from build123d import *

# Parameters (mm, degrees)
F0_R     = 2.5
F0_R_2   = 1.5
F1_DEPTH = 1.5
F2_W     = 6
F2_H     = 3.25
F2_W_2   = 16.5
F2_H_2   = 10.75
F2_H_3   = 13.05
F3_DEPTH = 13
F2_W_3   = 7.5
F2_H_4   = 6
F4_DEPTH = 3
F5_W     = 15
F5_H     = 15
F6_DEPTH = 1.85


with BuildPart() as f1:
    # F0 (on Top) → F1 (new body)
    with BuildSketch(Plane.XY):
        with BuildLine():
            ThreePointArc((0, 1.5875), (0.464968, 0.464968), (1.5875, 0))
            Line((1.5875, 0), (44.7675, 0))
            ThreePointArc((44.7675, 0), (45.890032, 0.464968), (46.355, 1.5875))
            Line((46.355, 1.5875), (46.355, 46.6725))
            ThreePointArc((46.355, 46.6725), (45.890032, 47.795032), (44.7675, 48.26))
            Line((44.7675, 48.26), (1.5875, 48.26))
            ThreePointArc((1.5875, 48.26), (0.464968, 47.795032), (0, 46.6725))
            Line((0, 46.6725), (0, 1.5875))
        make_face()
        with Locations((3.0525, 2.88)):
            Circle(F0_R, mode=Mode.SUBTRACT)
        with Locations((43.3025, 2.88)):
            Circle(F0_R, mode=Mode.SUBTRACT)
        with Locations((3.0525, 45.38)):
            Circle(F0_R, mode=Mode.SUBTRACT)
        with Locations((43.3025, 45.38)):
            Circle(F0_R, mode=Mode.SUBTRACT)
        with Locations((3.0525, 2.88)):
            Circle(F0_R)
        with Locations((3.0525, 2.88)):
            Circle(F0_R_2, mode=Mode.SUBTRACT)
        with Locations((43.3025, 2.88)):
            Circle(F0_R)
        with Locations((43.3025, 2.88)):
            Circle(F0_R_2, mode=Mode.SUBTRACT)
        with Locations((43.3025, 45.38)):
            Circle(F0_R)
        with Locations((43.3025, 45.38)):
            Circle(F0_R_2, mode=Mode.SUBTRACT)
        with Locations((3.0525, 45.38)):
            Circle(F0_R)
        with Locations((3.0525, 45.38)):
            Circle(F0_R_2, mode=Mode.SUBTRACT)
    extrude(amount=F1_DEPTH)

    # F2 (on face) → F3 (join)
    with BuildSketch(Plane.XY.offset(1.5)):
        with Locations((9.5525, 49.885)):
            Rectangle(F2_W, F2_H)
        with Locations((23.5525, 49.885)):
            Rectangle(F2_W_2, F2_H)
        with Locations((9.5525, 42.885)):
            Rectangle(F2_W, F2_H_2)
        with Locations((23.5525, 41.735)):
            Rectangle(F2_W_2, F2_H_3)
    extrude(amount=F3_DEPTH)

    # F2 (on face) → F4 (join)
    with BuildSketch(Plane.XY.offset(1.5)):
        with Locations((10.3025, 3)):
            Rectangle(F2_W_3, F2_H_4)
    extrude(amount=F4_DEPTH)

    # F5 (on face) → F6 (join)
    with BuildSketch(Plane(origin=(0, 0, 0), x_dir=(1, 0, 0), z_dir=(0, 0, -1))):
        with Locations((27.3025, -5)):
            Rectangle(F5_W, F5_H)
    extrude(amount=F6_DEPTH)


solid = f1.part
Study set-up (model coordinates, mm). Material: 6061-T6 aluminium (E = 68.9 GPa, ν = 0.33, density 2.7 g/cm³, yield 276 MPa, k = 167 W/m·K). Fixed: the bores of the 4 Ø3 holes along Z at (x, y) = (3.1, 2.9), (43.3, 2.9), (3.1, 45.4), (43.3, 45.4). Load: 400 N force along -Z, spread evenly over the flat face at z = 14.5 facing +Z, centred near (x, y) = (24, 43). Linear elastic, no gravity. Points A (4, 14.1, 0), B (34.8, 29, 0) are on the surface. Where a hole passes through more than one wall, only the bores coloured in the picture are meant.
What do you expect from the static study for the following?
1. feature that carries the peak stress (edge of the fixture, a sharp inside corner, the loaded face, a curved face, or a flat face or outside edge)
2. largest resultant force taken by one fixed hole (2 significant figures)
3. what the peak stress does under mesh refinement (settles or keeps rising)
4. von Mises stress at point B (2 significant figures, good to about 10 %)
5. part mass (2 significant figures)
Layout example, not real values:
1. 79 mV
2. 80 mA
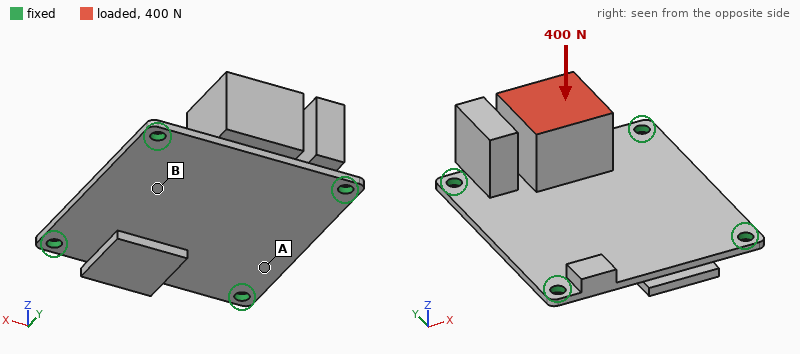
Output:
1. edge of the fixture
2. 220 N
3. keeps rising
4. 30 MPa
5. 23 g
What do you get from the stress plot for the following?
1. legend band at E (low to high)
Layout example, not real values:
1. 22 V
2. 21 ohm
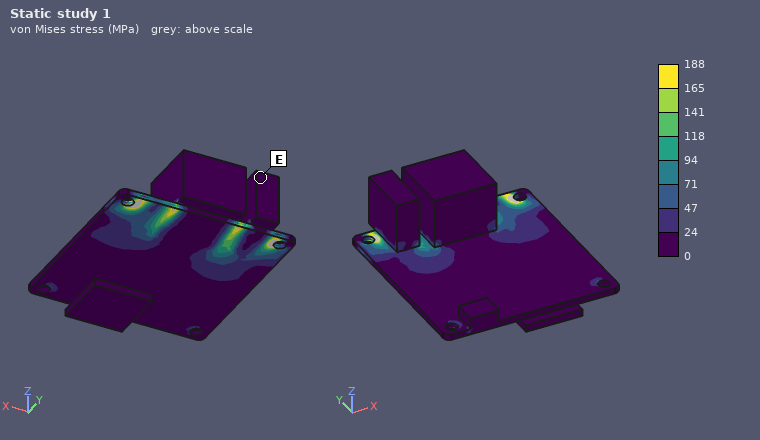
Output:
1. 0 to 24 MPa
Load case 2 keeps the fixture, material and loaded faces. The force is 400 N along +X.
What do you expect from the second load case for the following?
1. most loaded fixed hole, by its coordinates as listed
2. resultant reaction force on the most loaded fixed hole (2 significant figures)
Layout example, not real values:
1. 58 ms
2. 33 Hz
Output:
1. (3.1, 45.4)
2. 260 N
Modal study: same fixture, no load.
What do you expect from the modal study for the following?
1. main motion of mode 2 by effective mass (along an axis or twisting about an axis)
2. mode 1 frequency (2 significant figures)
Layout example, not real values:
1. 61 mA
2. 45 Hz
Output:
1. along Z
2. 2300 Hz
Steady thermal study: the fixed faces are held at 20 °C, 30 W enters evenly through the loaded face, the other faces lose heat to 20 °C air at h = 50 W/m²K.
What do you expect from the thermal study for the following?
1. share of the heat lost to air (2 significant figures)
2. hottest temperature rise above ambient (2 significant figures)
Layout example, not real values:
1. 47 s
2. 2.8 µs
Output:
1. 19 %
2. 46 K
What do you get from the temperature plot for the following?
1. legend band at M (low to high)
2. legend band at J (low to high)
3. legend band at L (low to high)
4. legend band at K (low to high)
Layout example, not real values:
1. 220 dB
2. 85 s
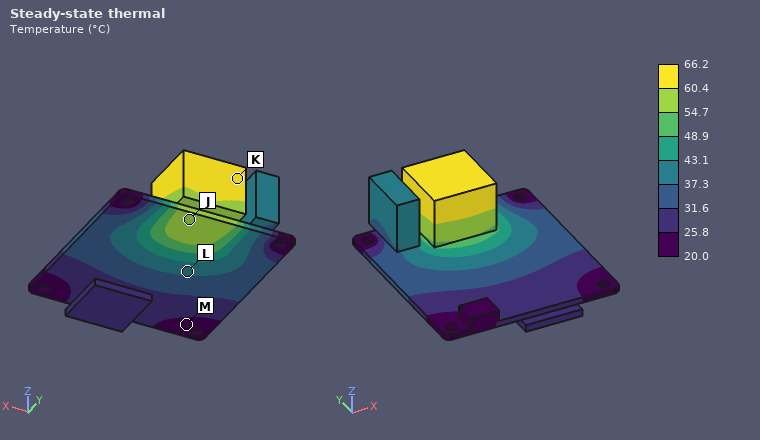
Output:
1. 20.0 to 25.8 °C
2. 54.7 to 60.4 °C
3. 37.3 to 43.1 °C
4. 60.4 to 66.2 °C
